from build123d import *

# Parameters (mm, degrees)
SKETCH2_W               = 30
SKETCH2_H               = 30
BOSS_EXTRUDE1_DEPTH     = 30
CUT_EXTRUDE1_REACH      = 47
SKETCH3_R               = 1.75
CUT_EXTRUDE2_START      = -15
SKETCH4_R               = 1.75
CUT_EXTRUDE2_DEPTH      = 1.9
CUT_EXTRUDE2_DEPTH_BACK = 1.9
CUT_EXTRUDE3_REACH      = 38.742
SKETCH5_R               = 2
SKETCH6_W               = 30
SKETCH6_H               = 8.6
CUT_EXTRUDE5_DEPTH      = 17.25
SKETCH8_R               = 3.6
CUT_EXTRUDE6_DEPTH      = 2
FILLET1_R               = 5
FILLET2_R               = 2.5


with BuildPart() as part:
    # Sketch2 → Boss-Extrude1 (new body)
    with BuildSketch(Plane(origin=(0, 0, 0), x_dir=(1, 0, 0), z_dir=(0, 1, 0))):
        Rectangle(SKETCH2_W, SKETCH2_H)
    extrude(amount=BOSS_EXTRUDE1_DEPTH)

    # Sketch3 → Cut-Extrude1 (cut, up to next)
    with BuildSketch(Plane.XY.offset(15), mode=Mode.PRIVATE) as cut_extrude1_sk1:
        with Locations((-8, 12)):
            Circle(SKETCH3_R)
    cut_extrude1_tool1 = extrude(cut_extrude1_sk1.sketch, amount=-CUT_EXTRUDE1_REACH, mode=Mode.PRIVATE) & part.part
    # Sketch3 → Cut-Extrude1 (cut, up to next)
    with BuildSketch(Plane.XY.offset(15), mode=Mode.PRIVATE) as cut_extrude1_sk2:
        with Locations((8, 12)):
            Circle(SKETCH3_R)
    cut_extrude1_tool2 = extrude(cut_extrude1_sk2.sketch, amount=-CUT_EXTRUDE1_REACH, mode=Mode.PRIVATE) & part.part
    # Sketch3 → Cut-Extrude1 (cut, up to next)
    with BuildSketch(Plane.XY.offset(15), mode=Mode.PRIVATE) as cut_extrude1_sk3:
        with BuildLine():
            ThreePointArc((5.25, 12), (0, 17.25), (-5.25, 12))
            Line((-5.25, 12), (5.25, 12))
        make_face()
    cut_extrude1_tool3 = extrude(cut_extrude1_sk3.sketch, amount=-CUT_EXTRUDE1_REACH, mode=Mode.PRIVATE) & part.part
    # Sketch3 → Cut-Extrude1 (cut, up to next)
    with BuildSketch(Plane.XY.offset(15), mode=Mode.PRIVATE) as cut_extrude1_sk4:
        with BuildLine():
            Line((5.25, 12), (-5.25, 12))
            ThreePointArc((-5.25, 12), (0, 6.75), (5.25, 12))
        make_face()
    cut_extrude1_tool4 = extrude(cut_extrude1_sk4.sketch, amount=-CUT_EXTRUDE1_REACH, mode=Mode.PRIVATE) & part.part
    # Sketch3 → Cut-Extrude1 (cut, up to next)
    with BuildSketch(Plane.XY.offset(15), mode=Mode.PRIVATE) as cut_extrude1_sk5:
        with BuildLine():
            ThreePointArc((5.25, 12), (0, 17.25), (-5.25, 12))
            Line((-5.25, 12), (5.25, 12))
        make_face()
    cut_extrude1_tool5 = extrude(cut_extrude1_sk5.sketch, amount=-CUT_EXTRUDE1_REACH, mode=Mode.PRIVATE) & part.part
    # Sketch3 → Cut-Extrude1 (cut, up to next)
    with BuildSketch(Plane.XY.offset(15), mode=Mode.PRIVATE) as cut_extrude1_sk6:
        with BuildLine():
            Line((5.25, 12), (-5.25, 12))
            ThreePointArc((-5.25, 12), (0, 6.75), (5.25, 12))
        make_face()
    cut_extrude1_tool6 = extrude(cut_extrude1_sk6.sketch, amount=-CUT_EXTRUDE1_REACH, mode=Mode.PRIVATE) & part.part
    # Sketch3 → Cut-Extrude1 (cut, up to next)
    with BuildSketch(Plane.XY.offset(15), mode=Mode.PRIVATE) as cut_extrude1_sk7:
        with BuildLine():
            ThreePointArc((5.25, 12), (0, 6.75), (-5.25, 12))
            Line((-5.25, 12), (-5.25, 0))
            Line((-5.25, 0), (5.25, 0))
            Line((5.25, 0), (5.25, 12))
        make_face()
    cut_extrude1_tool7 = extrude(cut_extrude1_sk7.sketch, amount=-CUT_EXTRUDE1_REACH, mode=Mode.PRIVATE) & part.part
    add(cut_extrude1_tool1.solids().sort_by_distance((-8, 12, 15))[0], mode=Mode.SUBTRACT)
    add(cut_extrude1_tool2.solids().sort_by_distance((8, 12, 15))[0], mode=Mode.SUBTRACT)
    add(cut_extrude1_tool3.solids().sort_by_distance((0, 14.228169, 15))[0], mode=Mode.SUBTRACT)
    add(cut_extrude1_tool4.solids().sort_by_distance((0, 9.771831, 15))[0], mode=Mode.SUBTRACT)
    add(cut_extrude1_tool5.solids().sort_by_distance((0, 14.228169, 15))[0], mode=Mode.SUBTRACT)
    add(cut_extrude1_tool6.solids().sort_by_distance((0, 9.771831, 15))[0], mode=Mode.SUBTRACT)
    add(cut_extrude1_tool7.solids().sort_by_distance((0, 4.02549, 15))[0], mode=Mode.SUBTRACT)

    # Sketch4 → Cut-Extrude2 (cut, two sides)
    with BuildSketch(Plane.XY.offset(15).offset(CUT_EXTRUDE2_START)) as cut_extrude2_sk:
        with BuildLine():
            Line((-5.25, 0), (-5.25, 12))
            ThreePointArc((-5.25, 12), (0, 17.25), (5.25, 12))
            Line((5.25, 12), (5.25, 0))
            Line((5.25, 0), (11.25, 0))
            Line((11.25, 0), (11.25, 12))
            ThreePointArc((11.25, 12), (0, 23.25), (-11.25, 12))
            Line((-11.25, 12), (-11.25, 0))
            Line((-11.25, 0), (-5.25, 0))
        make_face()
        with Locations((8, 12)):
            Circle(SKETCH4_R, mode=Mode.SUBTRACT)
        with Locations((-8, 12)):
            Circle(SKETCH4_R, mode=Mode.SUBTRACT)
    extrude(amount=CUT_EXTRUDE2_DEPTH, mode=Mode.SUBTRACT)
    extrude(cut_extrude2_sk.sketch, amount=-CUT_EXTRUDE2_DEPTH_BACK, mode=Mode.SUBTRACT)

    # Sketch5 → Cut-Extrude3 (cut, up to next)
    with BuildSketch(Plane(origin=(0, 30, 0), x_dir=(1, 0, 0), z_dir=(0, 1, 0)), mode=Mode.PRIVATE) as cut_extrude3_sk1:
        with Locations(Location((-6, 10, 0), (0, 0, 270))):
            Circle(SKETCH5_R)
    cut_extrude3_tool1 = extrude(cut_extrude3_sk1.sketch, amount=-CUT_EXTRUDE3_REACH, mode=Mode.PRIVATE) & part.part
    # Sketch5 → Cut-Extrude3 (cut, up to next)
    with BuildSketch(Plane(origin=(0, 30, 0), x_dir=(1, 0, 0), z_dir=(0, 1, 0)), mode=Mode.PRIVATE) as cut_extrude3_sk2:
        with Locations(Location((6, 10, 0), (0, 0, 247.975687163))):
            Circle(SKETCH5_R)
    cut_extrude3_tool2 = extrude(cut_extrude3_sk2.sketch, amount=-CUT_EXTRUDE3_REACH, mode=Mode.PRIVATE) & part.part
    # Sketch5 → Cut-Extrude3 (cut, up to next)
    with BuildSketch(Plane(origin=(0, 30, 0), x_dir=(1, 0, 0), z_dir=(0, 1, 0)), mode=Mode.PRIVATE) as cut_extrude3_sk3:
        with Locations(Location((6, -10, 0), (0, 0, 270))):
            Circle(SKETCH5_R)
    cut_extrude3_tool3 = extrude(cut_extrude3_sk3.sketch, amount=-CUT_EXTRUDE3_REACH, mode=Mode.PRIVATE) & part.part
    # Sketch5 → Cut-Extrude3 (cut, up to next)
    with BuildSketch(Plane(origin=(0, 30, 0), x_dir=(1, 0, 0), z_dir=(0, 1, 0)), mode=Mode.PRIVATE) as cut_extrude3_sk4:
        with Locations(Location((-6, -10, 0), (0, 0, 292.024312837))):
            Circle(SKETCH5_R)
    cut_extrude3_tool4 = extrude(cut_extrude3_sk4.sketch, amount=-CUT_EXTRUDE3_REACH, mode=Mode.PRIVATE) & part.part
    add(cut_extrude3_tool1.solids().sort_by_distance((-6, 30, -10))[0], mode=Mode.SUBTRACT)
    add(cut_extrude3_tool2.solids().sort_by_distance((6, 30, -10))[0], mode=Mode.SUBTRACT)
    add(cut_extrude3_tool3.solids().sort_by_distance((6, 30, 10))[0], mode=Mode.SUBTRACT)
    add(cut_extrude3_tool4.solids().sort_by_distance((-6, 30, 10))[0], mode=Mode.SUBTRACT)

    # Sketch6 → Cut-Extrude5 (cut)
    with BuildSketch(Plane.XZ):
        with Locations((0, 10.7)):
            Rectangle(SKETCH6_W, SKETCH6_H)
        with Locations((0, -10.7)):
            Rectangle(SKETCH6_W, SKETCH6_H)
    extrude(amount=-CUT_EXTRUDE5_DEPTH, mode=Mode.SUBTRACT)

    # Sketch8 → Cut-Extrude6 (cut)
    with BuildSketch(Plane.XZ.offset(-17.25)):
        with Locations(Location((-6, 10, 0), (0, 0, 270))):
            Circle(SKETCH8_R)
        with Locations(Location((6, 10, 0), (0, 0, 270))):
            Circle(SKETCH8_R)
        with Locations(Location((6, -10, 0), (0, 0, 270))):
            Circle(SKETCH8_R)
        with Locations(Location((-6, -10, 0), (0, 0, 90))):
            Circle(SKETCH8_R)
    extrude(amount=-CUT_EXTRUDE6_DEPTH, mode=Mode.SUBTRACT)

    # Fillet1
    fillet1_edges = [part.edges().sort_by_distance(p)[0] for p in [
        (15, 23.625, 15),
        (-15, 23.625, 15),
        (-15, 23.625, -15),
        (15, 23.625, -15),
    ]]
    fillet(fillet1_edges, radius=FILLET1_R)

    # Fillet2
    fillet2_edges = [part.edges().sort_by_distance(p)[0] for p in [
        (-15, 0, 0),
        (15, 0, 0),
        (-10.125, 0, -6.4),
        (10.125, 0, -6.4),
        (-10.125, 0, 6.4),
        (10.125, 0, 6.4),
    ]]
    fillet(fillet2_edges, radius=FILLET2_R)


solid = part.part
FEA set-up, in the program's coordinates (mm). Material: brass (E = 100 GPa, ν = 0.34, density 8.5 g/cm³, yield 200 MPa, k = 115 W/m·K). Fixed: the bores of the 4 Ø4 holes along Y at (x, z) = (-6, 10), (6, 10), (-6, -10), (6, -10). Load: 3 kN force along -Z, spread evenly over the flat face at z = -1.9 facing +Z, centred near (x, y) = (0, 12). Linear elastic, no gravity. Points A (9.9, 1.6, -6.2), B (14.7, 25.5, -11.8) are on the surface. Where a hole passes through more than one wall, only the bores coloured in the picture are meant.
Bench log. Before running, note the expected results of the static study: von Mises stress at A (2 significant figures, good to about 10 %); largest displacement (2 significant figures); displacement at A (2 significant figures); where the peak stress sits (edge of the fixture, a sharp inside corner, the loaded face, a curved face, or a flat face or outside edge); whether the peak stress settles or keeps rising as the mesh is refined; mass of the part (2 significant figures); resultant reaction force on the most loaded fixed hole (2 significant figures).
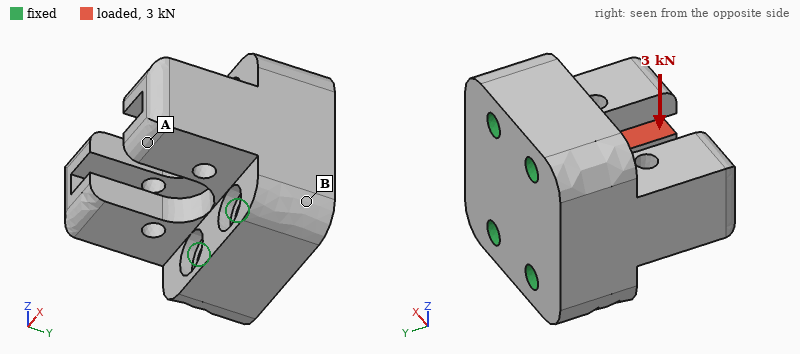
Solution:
27 MPa
43 µm
29 µm
a sharp inside corner
keeps rising
110 g
1.3 kN
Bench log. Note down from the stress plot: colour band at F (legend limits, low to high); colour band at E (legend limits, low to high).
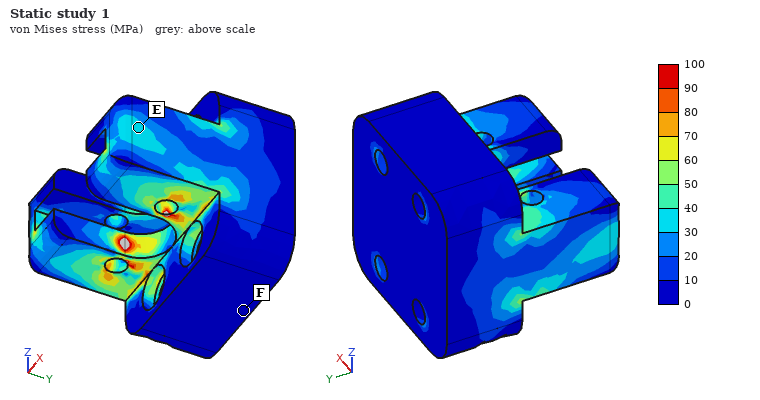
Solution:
0 to 10 MPa
30 to 40 MPa
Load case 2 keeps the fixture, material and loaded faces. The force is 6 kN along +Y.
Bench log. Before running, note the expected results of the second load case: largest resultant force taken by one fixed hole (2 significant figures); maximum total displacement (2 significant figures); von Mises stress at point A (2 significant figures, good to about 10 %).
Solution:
1.9 kN
28 µm
35 MPa
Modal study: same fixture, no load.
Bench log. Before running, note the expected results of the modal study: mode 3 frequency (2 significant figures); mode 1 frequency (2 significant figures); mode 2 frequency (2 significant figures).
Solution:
11 kHz
11 kHz
11 kHz
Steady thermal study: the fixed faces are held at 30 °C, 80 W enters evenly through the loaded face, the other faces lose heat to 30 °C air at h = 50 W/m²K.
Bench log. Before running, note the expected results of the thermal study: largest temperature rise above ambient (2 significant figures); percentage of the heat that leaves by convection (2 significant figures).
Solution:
51 K
3.9 %
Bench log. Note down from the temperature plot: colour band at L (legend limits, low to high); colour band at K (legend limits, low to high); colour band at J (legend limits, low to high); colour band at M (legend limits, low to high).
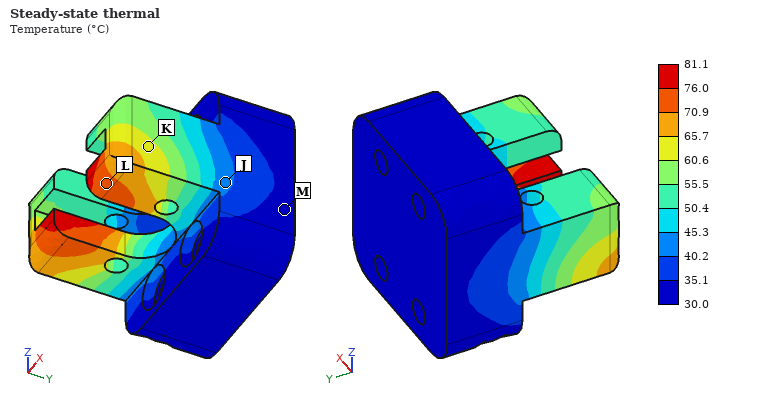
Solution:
70.9 to 76.0 °C
60.6 to 65.7 °C
40.2 to 45.3 °C
30.0 to 35.1 °C
